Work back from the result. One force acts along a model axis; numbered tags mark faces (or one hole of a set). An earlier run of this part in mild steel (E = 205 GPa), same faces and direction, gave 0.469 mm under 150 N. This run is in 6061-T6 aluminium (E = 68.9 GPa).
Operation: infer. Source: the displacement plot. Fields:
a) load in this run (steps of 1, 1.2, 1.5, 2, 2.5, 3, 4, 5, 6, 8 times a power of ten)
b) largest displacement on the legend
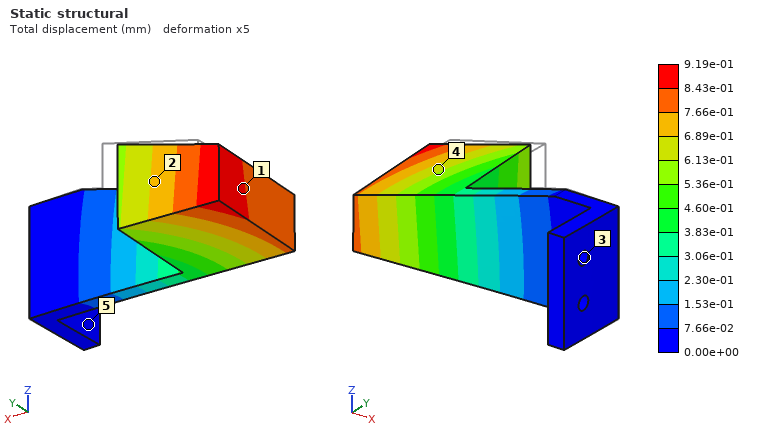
100 N
9.19e-01 mm
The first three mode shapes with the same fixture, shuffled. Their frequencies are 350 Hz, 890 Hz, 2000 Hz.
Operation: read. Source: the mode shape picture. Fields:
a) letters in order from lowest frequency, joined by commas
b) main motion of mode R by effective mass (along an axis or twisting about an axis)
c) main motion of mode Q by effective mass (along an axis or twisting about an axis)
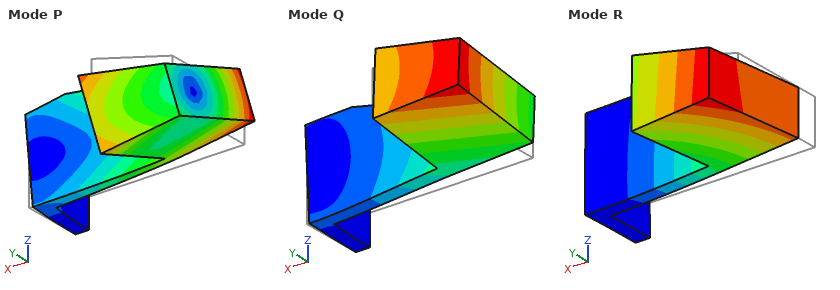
R, Q, P
along Y
along Z
